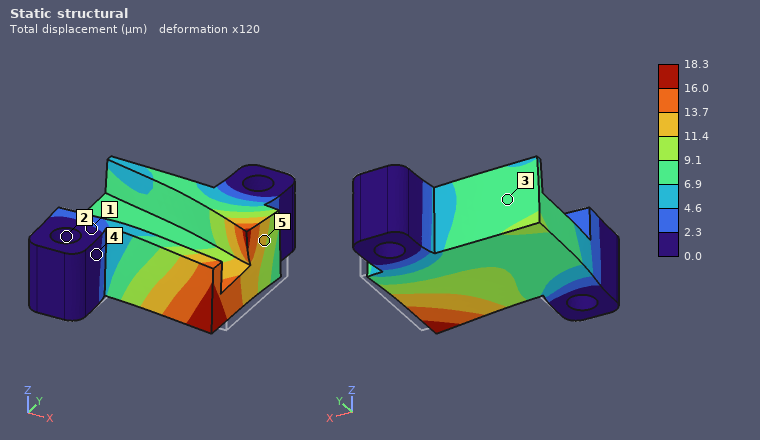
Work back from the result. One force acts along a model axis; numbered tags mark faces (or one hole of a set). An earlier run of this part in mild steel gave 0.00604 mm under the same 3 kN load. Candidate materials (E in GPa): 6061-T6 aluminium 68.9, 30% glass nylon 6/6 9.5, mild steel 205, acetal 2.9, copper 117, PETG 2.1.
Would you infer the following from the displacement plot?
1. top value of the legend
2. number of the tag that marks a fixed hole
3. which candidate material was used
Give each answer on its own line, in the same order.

18.3 µm
2
6061-T6 aluminium
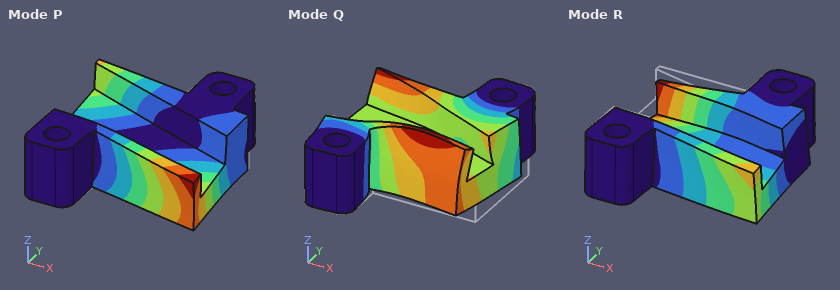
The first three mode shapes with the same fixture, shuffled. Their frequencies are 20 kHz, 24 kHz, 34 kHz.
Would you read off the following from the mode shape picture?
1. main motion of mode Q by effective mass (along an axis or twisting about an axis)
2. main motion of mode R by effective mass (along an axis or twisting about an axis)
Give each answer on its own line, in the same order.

along X
along Z
